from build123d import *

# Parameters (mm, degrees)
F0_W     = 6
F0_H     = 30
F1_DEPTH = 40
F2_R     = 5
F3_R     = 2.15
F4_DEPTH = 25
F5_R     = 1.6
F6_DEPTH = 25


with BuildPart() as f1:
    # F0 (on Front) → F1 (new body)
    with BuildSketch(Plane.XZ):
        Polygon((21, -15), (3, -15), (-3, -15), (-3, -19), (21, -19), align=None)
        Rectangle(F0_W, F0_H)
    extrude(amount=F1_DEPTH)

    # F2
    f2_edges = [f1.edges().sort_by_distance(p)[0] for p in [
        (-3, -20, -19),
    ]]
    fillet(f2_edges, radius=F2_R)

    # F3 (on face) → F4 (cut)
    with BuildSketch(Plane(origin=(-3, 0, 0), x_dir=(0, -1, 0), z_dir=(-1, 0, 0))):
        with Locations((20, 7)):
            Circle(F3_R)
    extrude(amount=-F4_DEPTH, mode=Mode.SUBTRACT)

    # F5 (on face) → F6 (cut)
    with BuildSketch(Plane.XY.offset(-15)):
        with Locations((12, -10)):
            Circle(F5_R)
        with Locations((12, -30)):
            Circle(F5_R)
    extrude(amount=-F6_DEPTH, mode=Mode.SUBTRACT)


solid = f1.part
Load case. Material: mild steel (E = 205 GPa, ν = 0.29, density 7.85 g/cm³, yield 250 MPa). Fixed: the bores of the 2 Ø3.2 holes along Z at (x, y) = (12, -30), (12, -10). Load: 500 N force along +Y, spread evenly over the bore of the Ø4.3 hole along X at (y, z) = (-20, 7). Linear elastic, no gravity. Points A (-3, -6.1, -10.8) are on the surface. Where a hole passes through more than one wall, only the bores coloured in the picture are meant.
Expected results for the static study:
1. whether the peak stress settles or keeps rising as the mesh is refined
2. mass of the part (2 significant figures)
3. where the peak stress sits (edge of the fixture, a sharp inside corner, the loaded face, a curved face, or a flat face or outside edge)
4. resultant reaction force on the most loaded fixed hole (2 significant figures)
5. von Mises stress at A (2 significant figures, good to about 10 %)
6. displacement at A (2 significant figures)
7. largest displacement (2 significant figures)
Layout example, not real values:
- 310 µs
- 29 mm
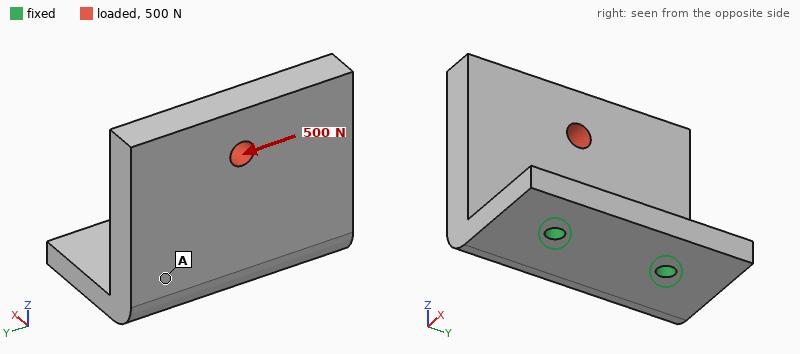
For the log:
- keeps rising
- 84 g
- edge of the fixture
- 610 N
- 14 MPa
- 8.9 µm
- 23 µm
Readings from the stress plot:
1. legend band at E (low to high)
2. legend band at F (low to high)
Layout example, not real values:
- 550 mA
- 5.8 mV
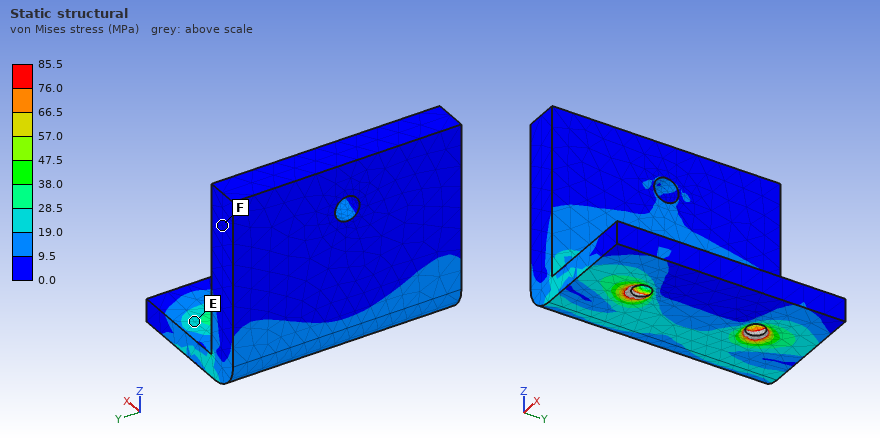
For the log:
- 19.0 to 28.5 MPa
- 0.0 to 9.5 MPa
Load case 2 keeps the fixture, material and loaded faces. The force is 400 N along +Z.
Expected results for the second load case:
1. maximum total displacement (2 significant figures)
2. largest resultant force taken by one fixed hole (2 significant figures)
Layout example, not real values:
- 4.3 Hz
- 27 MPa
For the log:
- 26 µm
- 200 N
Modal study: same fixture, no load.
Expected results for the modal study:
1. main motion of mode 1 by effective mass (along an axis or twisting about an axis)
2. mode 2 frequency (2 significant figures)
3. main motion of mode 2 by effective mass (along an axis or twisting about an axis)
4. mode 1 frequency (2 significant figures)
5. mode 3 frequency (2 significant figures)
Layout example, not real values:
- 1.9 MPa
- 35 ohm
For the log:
- along X
- 4200 Hz
- along Y
- 1900 Hz
- 7800 Hz
